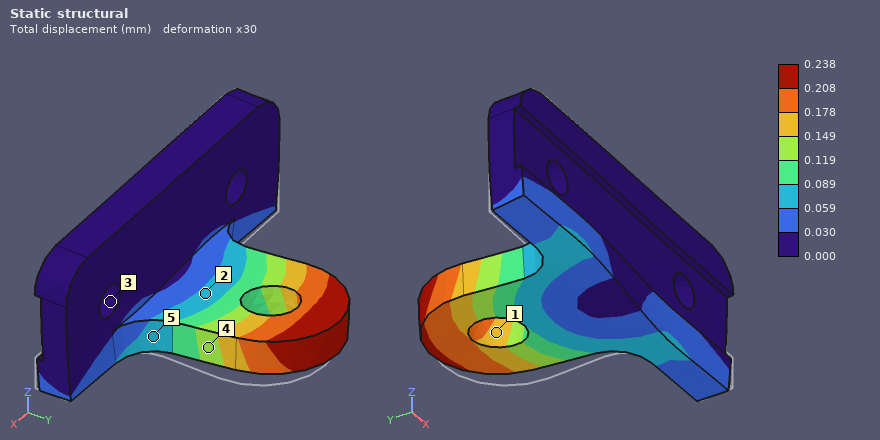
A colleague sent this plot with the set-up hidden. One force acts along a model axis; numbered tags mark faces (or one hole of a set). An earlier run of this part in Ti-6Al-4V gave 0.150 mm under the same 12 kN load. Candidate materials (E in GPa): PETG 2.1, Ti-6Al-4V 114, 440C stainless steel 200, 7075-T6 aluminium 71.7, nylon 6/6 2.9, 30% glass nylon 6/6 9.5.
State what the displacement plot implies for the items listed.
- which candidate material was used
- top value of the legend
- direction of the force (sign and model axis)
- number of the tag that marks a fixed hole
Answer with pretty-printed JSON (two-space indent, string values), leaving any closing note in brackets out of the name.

{
  "which candidate material was used": "7075-T6 aluminium",
  "top value of the legend": "0.238 mm",
  "direction of the force": "-X",
  "number of the tag that marks a fixed hole": "3"
}
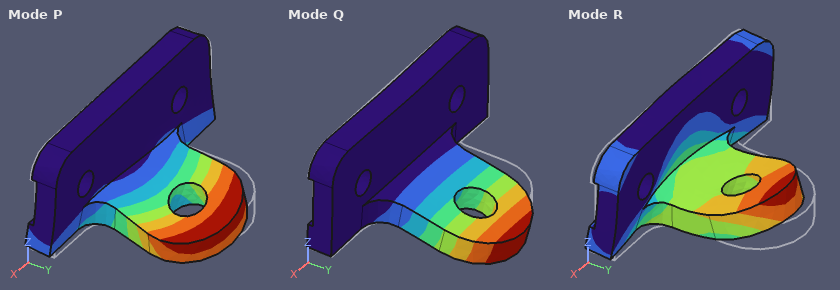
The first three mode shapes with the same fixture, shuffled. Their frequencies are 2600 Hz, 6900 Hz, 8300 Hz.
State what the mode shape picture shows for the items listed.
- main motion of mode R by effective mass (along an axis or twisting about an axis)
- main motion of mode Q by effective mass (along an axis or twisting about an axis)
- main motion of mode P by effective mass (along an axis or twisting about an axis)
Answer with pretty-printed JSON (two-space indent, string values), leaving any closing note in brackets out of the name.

{
  "main motion of mode R by effective mass": "along Y",
  "main motion of mode Q by effective mass": "along Z",
  "main motion of mode P by effective mass": "along X"
}
